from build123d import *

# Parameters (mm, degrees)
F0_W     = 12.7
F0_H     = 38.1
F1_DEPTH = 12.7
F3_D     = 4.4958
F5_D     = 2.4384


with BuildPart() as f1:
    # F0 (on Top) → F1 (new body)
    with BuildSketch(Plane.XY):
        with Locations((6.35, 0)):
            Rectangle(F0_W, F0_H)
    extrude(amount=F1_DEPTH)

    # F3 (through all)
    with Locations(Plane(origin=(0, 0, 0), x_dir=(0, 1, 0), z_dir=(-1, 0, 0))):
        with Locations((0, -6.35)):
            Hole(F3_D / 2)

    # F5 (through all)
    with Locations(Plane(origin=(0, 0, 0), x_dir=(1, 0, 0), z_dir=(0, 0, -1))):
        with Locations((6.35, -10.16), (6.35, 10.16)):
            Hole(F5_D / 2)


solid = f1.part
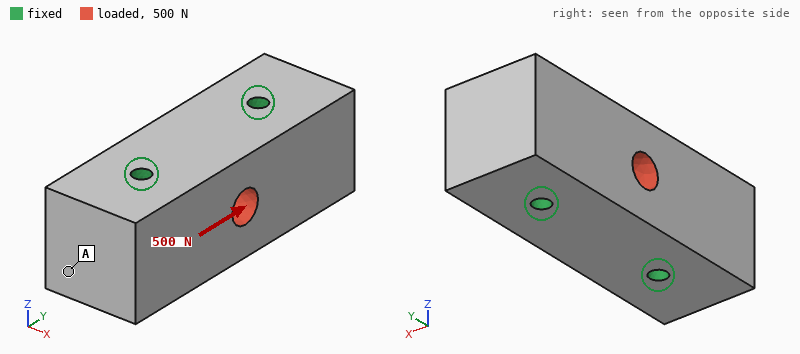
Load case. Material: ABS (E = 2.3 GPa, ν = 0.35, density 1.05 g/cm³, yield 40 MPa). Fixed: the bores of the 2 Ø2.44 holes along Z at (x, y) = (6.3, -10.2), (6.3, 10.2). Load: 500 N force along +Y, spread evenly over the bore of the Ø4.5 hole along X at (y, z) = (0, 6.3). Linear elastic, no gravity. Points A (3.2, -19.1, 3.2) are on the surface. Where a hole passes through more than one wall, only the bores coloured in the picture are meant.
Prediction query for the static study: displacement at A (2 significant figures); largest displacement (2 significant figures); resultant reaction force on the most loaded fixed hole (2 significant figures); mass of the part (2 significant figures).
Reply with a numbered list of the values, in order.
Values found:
1. 2.1 µm
2. 10 µm
3. 250 N
4. 6.1 g
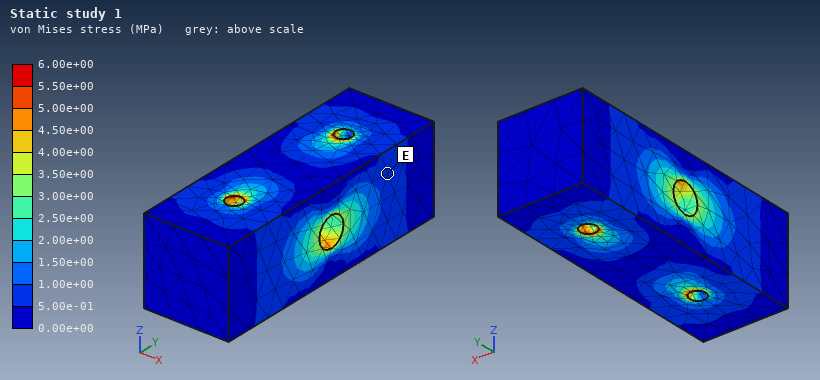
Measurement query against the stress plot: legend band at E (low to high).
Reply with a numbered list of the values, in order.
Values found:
1. 5.00e-01 to 1.00e+00 MPa
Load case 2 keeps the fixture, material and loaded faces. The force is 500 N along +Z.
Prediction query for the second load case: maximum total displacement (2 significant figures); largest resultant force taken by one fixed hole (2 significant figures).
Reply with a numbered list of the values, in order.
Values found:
1. 29 µm
2. 250 N
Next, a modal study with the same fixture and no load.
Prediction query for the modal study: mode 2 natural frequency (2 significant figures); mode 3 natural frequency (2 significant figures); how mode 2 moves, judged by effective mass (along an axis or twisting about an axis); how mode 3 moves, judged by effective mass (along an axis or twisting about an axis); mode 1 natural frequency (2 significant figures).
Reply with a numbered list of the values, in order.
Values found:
1. 13 kHz
2. 17 kHz
3. twisting about Z
4. twisting about X
5. 12 kHz
